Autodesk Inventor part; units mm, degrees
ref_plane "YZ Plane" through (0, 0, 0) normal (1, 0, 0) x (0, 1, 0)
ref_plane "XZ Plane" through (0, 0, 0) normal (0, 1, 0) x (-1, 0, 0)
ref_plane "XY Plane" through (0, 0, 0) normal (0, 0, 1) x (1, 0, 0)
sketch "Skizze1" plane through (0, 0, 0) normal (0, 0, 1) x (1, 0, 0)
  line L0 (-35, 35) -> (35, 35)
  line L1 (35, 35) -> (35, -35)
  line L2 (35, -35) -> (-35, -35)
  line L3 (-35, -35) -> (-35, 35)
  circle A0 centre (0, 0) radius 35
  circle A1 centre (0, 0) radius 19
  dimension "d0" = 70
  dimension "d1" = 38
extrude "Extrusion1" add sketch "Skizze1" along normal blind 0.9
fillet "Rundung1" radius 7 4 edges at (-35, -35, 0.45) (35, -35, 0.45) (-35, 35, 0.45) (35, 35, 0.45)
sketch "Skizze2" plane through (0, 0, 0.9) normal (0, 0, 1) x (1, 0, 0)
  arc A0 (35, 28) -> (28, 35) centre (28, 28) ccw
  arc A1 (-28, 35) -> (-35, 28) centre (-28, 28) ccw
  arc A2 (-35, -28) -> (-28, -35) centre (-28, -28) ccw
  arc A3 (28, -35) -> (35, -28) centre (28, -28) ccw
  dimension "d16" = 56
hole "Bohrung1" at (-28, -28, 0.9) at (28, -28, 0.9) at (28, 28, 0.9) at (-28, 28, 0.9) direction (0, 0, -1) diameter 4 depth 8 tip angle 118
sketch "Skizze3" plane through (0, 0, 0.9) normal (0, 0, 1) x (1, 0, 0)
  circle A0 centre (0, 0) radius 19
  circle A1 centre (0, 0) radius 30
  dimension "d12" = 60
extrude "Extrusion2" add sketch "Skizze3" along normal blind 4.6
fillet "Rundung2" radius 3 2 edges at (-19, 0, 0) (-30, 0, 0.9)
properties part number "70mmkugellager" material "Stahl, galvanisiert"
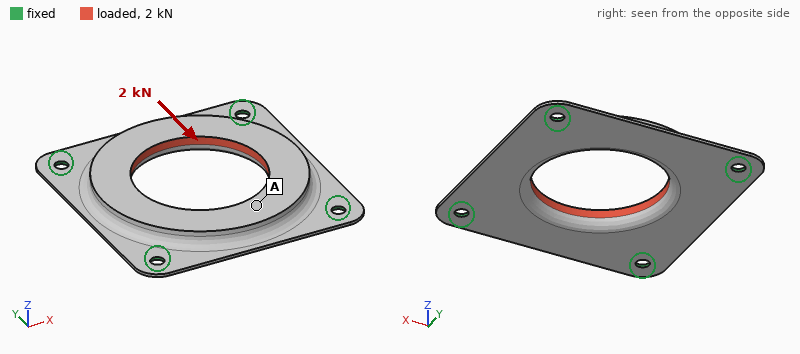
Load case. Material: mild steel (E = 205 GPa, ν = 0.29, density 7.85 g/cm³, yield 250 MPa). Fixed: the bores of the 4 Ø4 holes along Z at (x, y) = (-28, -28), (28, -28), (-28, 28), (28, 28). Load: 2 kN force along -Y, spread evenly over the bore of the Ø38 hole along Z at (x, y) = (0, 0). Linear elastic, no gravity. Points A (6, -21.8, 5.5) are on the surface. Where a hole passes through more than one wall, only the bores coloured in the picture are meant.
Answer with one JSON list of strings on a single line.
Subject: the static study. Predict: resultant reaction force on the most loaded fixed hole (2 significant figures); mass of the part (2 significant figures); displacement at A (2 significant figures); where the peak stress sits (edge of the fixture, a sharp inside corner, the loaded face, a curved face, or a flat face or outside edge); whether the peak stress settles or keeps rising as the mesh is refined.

["530 N", "88 g", "12 µm", "edge of the fixture", "keeps rising"]
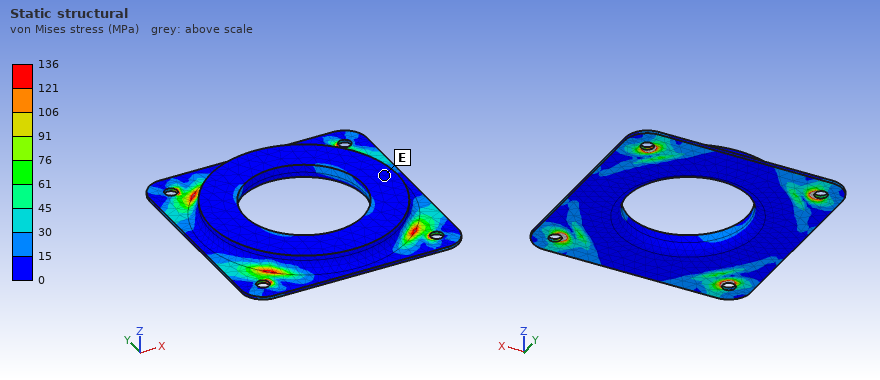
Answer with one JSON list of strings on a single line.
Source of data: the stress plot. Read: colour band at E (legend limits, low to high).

["0 to 15 MPa"]
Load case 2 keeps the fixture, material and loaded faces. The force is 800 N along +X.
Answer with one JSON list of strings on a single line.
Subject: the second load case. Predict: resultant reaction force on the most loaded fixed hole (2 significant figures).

["210 N"]
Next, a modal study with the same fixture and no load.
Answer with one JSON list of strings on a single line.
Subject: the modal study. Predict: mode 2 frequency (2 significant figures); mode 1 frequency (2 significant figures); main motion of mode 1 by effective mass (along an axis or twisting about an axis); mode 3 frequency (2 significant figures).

["3200 Hz", "2400 Hz", "along Z", "3200 Hz"]
